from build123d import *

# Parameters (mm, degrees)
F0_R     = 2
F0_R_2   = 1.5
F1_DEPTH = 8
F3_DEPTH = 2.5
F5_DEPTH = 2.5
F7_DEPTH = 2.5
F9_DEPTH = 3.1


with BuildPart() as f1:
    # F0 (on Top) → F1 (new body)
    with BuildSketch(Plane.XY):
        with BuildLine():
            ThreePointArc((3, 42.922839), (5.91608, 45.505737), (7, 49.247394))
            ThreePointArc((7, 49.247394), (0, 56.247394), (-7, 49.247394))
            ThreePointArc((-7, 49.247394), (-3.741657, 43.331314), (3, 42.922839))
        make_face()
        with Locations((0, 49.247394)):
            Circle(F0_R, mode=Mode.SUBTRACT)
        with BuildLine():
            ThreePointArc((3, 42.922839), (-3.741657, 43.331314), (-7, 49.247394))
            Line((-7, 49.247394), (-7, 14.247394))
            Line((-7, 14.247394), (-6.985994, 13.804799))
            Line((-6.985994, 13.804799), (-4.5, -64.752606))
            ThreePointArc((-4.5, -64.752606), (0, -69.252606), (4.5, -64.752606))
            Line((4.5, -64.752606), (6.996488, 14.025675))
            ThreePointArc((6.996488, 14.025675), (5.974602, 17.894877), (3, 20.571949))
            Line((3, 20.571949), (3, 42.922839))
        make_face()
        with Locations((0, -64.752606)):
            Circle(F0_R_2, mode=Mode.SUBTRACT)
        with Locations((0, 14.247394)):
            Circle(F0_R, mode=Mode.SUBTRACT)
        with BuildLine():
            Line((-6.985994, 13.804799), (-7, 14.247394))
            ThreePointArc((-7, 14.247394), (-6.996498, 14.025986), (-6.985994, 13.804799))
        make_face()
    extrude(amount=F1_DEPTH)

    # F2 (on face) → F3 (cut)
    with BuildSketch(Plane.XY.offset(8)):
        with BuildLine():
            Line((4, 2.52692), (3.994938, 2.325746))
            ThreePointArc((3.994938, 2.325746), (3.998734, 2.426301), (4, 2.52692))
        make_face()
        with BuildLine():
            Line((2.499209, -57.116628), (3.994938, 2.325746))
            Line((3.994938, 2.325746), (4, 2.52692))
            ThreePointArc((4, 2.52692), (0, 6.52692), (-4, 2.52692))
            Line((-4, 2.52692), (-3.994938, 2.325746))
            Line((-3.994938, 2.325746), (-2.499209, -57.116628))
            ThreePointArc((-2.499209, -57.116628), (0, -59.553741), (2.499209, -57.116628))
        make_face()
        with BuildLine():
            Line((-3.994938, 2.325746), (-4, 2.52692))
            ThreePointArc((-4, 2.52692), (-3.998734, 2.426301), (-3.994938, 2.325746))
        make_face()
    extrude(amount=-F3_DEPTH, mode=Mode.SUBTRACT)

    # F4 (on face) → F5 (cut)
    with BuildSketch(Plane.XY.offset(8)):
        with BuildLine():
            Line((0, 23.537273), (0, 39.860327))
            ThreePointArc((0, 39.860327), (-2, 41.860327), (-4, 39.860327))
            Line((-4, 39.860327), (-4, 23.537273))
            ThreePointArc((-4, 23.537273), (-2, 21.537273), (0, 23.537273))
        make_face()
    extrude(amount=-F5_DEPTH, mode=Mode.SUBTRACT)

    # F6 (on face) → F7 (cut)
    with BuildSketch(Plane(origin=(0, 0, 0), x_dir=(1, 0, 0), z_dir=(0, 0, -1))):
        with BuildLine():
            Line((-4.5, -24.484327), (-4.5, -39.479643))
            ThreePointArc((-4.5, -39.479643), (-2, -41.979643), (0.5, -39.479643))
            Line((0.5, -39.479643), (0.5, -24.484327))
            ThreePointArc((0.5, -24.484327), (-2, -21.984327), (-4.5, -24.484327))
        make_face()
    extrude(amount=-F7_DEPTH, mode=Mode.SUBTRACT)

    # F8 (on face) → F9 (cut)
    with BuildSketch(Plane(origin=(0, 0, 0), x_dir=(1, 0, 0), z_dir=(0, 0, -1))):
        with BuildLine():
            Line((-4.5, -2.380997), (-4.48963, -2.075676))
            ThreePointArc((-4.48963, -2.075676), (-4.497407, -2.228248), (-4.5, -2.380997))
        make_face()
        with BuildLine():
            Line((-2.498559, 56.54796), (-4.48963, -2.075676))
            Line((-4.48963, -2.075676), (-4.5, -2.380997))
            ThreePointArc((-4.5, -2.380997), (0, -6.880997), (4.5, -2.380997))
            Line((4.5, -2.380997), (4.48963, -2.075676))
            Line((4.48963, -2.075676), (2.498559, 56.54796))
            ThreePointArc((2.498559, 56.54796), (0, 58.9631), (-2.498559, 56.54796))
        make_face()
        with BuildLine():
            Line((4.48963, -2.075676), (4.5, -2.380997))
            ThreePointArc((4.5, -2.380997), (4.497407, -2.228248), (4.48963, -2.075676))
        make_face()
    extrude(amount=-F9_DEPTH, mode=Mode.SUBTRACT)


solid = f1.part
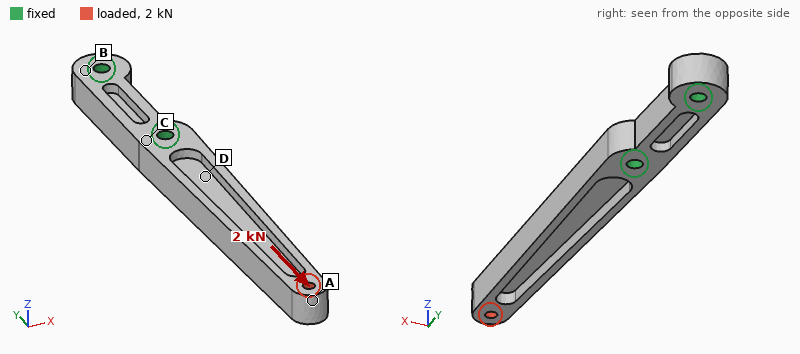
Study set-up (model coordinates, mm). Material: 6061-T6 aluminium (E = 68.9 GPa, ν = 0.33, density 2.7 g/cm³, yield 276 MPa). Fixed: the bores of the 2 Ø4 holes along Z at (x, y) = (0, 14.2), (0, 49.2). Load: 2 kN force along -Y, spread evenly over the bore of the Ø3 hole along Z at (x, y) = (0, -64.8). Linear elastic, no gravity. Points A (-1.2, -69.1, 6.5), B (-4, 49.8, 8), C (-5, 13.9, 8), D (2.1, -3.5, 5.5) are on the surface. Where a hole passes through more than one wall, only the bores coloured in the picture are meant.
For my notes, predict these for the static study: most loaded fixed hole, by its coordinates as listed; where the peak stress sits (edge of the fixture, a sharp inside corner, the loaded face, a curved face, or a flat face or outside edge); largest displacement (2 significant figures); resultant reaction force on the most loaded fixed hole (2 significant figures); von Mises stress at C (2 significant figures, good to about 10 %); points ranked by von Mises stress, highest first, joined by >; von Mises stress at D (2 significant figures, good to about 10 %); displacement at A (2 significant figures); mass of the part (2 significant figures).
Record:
(0, 14.2)
the loaded face
88 µm
1.9 kN
10 MPa
D > A > C > B
33 MPa
83 µm
22 g
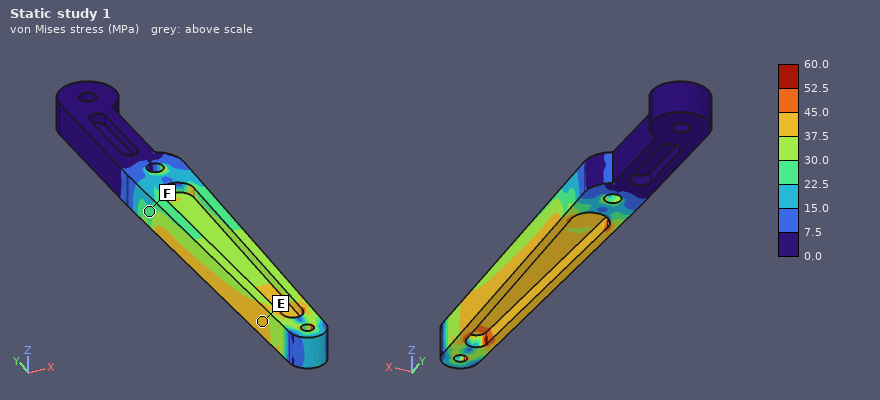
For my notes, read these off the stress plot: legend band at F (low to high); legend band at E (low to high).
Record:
22.5 to 30.0 MPa
37.5 to 45.0 MPa
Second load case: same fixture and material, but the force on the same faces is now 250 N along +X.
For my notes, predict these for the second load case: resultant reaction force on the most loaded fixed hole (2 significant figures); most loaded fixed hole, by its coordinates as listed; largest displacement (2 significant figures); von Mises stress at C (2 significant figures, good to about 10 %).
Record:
510 N
(0, 14.2)
0.69 mm
46 MPa
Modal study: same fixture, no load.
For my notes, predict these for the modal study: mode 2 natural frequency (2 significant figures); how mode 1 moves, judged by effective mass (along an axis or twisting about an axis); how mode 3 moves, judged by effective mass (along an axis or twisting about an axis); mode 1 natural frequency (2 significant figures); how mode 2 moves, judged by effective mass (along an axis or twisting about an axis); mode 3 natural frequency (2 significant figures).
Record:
1700 Hz
along Z
twisting about Y
880 Hz
along X
4300 Hz
